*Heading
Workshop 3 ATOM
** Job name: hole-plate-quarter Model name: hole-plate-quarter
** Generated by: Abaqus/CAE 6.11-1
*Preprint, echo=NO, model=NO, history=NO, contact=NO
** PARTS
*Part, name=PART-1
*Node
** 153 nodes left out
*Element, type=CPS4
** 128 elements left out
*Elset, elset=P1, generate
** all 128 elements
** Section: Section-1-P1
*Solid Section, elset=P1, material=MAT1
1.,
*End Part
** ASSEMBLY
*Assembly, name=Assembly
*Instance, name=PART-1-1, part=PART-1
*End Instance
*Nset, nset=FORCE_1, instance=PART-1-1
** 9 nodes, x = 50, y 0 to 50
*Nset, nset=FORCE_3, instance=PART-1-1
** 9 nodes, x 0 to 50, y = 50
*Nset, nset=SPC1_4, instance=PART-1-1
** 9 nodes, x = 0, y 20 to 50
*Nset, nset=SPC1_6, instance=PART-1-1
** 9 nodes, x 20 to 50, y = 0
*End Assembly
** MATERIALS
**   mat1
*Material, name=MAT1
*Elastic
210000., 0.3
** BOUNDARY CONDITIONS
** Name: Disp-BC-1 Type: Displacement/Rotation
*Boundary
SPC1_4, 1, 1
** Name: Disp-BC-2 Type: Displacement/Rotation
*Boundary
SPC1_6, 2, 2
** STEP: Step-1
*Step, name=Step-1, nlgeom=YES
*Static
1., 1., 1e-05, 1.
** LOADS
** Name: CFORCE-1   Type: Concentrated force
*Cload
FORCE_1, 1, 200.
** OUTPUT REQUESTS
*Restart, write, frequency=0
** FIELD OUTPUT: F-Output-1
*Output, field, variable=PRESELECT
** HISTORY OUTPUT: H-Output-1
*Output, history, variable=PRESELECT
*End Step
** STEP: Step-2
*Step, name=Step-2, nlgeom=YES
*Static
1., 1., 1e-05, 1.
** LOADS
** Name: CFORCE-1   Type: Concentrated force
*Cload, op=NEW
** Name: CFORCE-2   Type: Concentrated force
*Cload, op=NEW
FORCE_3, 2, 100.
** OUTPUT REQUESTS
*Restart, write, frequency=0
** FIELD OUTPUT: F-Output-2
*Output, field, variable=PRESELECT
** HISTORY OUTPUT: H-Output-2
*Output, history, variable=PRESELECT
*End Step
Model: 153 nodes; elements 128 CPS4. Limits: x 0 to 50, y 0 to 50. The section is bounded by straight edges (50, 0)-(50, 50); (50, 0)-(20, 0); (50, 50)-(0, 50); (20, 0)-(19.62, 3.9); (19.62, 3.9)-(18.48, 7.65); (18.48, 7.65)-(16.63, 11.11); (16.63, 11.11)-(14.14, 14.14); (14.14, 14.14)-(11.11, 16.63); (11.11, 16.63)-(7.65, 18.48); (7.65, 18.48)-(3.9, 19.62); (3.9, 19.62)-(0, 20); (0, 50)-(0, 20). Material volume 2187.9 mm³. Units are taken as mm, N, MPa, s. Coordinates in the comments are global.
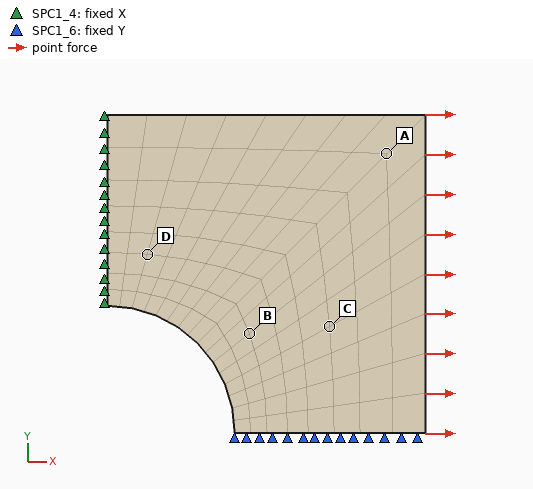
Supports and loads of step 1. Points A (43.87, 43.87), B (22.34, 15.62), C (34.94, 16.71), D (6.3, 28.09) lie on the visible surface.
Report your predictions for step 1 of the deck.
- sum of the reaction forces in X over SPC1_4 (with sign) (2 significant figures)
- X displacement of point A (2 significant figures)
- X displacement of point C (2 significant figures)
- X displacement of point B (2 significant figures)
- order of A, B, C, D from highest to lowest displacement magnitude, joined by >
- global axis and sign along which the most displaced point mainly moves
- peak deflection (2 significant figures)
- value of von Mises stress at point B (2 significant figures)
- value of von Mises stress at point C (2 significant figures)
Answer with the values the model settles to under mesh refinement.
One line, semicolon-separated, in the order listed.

-1800 N; 0.0075 mm; 0.014 mm; 0.012 mm; C > B > D > A; +X; 0.023 mm; 60 MPa; 48 MPa
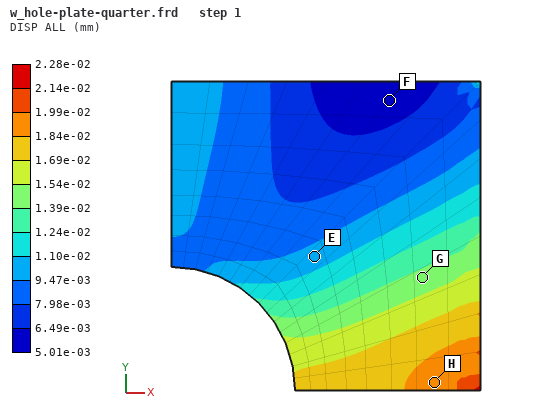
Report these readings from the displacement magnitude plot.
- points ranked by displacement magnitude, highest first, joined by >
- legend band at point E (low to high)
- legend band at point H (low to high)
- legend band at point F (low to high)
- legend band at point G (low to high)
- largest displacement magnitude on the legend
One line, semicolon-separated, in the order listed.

H > G > E > F; 9.47e-03 to 1.10e-02 mm; 1.84e-02 to 1.99e-02 mm; 5.01e-03 to 6.49e-03 mm; 1.39e-02 to 1.54e-02 mm; 2.28e-02 mm
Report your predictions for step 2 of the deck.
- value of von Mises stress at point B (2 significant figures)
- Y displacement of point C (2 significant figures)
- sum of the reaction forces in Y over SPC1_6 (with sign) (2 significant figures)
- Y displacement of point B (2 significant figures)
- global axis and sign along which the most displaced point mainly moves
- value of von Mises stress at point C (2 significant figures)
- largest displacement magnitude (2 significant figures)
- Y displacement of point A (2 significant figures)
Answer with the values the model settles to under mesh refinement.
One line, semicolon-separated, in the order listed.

35 MPa; 0.0020 mm; -900 N; 0.0035 mm; +Y; 27 MPa; 0.011 mm; 0.0037 mm
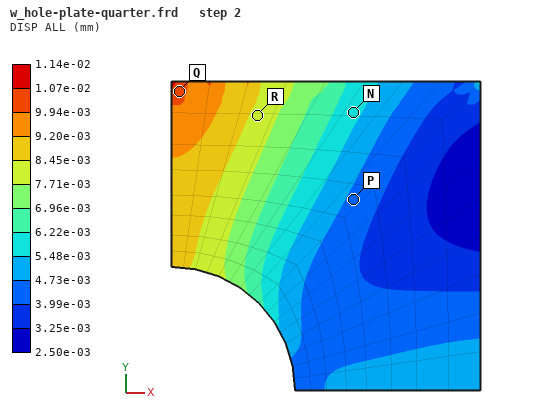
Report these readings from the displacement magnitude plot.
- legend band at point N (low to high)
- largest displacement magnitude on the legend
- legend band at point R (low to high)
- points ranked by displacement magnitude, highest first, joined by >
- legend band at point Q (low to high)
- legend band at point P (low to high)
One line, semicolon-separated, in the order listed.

5.48e-03 to 6.22e-03 mm; 1.14e-02 mm; 7.71e-03 to 8.45e-03 mm; Q > R > N > P; 9.94e-03 to 1.07e-02 mm; 3.99e-03 to 4.73e-03 mm
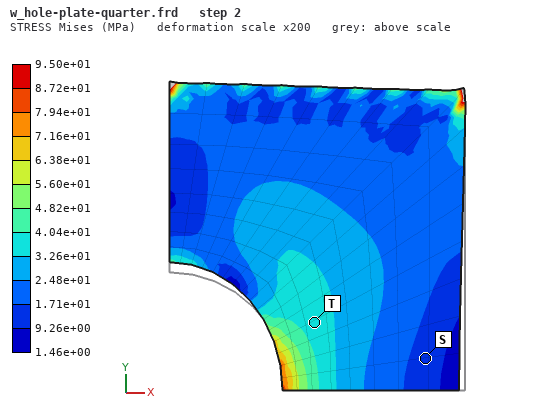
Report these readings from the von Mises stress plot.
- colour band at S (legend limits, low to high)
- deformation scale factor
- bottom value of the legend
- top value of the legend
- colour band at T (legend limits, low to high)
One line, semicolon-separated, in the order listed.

9.26e+00 to 1.71e+01 MPa; 200; 1.46e+00 MPa; 9.50e+01 MPa; 3.26e+01 to 4.04e+01 MPa
